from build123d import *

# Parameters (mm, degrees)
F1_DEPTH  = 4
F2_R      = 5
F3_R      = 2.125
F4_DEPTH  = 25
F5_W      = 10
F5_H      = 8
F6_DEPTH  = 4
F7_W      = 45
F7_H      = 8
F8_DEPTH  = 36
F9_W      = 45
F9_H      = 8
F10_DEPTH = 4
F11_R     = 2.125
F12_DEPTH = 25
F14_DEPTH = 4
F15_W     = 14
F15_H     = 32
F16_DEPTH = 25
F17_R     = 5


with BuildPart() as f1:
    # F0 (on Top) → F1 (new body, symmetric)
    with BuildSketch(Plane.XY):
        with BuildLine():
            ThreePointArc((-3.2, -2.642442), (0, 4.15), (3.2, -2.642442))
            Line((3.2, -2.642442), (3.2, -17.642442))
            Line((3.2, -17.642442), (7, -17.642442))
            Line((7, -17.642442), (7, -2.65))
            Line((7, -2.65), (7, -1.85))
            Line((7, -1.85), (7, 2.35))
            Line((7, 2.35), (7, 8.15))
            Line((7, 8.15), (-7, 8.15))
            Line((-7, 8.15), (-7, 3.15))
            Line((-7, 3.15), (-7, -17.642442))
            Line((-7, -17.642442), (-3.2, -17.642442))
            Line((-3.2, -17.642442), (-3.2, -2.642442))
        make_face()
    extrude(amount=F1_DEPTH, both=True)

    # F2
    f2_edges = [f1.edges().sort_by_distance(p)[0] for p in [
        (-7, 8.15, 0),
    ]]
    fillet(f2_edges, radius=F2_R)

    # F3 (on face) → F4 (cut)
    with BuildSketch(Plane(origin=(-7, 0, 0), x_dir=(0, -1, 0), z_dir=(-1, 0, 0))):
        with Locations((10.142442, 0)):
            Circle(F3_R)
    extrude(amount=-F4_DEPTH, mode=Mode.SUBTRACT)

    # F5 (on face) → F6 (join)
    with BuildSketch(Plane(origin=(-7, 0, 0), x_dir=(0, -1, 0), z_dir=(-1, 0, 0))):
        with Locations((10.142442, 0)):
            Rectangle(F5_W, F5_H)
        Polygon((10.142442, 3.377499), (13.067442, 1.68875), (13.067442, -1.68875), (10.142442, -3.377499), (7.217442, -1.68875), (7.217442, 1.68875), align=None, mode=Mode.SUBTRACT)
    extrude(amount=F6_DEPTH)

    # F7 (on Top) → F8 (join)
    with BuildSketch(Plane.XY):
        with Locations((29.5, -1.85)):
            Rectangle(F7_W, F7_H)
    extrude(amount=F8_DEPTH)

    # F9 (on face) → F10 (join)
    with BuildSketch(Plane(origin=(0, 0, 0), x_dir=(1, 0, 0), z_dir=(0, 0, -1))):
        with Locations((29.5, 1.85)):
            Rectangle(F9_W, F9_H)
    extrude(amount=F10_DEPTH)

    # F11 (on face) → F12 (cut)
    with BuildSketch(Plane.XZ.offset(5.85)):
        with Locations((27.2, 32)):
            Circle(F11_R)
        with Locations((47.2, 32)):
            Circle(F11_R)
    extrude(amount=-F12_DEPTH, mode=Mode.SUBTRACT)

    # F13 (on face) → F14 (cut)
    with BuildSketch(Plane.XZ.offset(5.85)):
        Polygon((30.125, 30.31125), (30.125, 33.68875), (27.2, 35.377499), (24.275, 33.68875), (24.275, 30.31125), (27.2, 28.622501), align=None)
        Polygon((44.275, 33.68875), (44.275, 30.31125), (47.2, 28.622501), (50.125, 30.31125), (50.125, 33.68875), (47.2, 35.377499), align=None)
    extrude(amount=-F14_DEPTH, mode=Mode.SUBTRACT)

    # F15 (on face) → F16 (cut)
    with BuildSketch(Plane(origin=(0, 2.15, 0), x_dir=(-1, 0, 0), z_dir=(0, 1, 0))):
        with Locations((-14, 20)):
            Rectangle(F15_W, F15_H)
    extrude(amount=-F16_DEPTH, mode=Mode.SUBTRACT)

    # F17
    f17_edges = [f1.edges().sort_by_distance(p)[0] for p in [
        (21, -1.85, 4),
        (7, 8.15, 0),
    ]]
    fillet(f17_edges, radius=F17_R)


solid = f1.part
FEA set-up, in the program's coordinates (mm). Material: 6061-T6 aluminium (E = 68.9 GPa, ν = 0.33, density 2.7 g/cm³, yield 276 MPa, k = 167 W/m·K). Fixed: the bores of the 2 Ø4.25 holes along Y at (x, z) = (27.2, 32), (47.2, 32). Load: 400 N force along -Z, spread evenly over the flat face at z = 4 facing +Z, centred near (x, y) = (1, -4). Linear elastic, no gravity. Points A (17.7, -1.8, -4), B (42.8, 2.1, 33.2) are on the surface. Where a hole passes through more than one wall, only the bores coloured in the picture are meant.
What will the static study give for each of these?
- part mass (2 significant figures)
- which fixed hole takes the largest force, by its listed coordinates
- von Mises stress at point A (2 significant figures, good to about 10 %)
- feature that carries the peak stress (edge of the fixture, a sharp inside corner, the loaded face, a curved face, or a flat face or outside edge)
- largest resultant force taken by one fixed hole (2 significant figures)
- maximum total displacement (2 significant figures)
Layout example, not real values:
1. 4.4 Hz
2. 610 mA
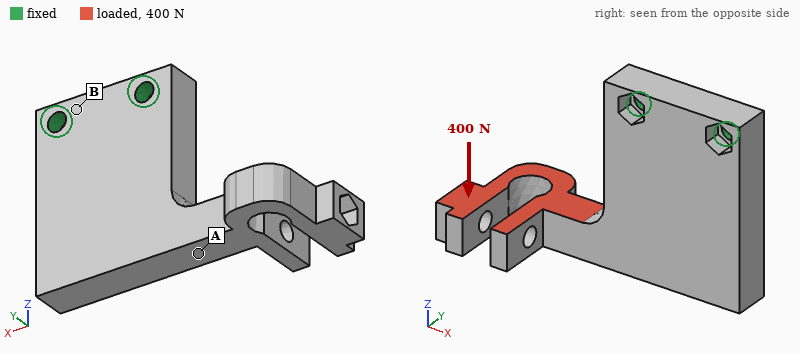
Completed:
1. 33 g
2. (27.2, 32)
3. 66 MPa
4. a curved face
5. 850 N
6. 0.38 mm
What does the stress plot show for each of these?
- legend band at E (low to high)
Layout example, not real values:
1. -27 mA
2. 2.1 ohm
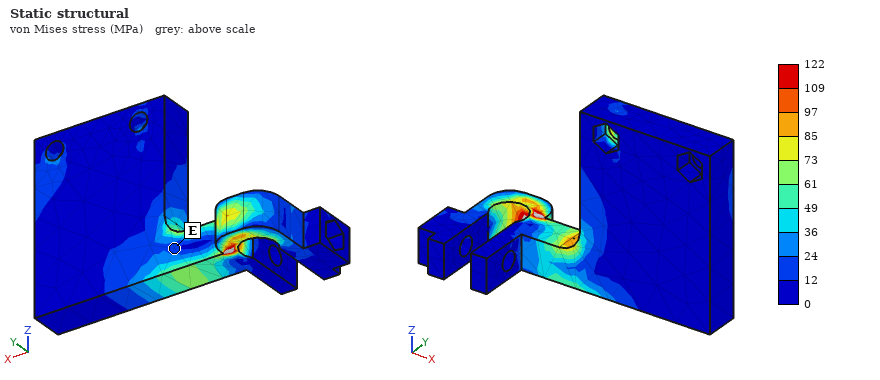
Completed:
1. 12 to 24 MPa
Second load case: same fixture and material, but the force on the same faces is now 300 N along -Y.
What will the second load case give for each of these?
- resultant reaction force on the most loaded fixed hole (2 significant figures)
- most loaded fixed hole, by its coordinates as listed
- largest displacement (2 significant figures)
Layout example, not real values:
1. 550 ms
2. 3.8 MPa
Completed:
1. 630 N
2. (27.2, 32)
3. 0.44 mm
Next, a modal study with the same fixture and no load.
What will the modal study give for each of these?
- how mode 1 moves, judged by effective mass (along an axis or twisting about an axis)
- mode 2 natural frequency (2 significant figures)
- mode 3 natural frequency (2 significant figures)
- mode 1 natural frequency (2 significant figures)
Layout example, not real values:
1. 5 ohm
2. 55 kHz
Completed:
1. along Y
2. 2600 Hz
3. 2900 Hz
4. 1900 Hz
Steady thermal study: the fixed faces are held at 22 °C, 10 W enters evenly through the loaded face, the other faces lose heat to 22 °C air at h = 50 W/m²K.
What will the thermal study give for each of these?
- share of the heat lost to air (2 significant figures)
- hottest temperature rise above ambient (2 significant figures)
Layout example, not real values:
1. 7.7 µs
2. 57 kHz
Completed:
1. 27 %
2. 36 K
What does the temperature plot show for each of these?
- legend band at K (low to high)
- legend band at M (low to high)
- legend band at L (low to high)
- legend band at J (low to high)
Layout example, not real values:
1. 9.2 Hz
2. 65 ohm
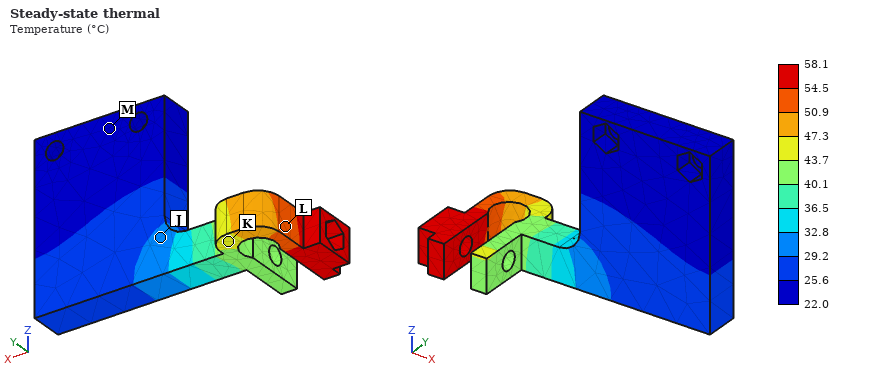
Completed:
1. 43.7 to 47.3 °C
2. 22.0 to 25.6 °C
3. 50.9 to 54.5 °C
4. 29.2 to 32.8 °C
